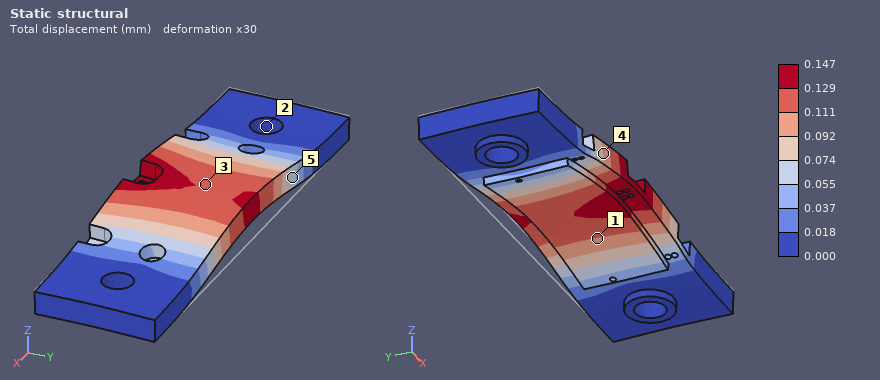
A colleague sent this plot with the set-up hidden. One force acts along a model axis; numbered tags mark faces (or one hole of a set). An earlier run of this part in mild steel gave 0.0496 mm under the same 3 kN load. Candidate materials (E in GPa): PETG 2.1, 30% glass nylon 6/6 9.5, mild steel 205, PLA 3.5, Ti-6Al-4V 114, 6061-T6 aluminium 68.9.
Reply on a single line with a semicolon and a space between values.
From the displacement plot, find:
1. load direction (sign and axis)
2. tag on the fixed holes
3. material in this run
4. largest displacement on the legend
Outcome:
+Z; 2; 6061-T6 aluminium; 0.147 mm
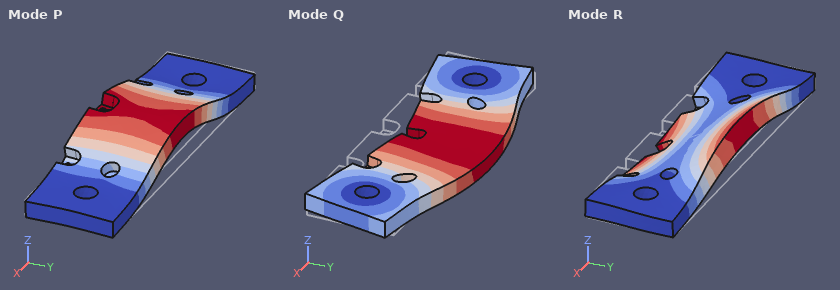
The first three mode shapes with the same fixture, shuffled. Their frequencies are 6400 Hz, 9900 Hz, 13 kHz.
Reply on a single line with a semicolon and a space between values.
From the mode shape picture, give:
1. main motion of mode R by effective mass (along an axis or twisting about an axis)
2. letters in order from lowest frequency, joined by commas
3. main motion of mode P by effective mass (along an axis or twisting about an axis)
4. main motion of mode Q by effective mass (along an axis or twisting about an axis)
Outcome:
twisting about X; P, R, Q; along Z; along Y
